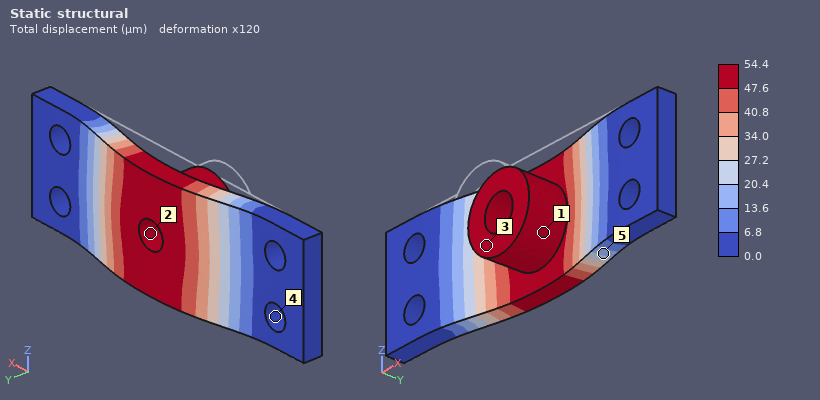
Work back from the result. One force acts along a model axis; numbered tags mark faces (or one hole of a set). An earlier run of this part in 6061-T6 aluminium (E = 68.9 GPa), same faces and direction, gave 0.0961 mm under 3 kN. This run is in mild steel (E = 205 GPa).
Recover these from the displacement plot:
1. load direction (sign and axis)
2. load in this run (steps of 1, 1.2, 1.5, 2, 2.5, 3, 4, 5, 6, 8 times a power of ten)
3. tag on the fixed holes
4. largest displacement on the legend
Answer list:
+Y
5 kN
4
54.4 µm
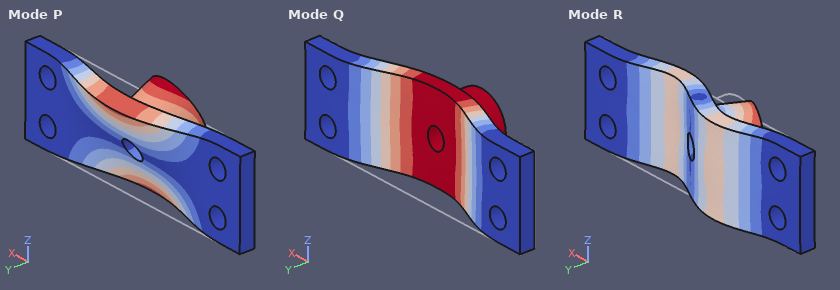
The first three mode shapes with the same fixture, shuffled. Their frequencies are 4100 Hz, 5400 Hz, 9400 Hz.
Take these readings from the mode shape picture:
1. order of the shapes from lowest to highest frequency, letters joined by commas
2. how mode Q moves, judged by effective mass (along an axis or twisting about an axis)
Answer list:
Q, P, R
along Y
